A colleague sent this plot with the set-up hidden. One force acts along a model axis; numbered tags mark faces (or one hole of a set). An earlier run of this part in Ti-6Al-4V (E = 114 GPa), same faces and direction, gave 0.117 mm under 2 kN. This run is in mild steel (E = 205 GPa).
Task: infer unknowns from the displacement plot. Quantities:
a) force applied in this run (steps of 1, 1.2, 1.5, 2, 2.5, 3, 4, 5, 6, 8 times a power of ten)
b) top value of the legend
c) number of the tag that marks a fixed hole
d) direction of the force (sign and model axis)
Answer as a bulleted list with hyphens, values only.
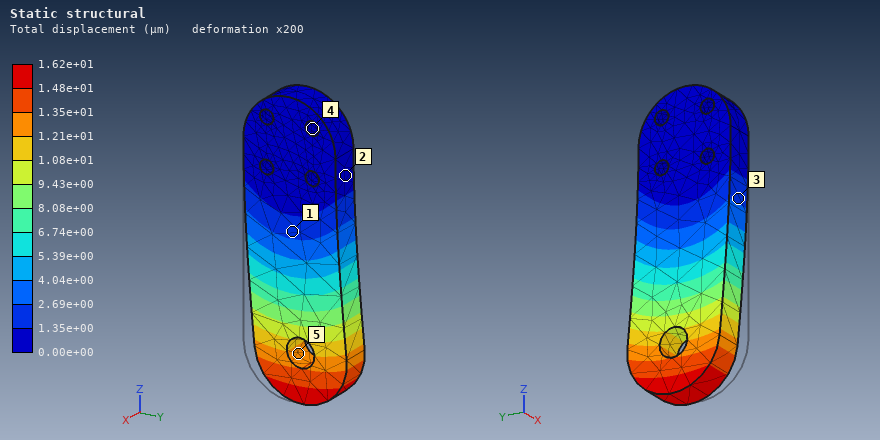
- 500 N
- 1.62e+01 µm
- 4
- +Y
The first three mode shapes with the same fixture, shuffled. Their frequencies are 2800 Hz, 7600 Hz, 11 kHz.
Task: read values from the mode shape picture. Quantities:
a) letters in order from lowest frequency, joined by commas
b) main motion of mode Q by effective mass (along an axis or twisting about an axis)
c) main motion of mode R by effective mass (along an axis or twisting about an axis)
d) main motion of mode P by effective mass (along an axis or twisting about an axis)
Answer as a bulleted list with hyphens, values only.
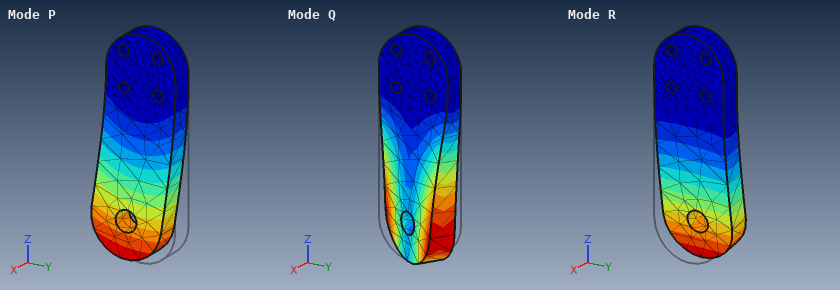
- R, P, Q
- twisting about Z
- along X
- along Y
